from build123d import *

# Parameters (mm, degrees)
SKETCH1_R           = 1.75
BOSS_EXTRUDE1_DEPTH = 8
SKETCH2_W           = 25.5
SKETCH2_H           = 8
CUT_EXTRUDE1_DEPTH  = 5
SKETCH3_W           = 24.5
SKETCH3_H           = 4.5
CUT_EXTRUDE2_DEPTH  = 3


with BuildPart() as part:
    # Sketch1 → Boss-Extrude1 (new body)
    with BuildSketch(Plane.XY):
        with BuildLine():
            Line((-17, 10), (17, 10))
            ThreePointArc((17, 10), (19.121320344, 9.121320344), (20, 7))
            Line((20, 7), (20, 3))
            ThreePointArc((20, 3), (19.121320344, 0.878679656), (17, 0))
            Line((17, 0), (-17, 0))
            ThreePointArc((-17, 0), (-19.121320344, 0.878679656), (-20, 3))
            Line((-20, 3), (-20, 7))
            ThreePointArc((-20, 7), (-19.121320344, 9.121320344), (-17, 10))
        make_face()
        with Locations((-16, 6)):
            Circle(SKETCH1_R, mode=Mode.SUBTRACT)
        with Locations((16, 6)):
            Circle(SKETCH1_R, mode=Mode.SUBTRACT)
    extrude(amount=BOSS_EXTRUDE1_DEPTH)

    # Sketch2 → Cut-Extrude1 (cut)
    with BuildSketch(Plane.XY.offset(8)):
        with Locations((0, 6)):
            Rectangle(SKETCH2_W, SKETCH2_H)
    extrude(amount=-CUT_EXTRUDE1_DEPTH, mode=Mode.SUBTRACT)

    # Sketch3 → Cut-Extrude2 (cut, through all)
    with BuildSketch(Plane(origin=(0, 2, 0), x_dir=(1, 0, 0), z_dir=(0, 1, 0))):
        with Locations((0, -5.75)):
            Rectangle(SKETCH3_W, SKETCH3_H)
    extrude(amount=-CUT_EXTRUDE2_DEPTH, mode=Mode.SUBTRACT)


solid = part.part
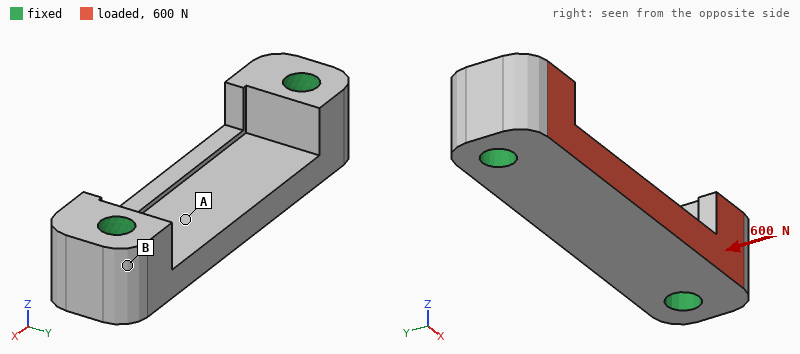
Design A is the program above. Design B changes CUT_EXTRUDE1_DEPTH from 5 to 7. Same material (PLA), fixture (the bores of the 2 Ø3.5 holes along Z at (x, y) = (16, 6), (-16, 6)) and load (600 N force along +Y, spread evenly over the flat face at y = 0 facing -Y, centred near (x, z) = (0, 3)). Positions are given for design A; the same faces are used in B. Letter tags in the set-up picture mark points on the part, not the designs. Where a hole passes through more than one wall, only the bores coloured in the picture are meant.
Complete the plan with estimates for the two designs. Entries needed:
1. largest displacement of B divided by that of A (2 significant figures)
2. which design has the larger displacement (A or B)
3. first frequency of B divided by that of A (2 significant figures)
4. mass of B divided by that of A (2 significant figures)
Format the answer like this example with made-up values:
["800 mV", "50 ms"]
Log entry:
["5.0", "B", "0.62", "0.77"]
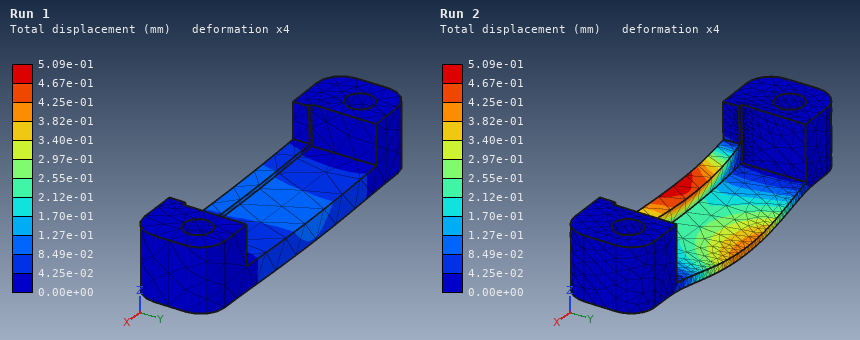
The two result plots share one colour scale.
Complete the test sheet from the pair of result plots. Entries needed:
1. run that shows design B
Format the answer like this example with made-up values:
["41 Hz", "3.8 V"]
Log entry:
["Run 2"]
